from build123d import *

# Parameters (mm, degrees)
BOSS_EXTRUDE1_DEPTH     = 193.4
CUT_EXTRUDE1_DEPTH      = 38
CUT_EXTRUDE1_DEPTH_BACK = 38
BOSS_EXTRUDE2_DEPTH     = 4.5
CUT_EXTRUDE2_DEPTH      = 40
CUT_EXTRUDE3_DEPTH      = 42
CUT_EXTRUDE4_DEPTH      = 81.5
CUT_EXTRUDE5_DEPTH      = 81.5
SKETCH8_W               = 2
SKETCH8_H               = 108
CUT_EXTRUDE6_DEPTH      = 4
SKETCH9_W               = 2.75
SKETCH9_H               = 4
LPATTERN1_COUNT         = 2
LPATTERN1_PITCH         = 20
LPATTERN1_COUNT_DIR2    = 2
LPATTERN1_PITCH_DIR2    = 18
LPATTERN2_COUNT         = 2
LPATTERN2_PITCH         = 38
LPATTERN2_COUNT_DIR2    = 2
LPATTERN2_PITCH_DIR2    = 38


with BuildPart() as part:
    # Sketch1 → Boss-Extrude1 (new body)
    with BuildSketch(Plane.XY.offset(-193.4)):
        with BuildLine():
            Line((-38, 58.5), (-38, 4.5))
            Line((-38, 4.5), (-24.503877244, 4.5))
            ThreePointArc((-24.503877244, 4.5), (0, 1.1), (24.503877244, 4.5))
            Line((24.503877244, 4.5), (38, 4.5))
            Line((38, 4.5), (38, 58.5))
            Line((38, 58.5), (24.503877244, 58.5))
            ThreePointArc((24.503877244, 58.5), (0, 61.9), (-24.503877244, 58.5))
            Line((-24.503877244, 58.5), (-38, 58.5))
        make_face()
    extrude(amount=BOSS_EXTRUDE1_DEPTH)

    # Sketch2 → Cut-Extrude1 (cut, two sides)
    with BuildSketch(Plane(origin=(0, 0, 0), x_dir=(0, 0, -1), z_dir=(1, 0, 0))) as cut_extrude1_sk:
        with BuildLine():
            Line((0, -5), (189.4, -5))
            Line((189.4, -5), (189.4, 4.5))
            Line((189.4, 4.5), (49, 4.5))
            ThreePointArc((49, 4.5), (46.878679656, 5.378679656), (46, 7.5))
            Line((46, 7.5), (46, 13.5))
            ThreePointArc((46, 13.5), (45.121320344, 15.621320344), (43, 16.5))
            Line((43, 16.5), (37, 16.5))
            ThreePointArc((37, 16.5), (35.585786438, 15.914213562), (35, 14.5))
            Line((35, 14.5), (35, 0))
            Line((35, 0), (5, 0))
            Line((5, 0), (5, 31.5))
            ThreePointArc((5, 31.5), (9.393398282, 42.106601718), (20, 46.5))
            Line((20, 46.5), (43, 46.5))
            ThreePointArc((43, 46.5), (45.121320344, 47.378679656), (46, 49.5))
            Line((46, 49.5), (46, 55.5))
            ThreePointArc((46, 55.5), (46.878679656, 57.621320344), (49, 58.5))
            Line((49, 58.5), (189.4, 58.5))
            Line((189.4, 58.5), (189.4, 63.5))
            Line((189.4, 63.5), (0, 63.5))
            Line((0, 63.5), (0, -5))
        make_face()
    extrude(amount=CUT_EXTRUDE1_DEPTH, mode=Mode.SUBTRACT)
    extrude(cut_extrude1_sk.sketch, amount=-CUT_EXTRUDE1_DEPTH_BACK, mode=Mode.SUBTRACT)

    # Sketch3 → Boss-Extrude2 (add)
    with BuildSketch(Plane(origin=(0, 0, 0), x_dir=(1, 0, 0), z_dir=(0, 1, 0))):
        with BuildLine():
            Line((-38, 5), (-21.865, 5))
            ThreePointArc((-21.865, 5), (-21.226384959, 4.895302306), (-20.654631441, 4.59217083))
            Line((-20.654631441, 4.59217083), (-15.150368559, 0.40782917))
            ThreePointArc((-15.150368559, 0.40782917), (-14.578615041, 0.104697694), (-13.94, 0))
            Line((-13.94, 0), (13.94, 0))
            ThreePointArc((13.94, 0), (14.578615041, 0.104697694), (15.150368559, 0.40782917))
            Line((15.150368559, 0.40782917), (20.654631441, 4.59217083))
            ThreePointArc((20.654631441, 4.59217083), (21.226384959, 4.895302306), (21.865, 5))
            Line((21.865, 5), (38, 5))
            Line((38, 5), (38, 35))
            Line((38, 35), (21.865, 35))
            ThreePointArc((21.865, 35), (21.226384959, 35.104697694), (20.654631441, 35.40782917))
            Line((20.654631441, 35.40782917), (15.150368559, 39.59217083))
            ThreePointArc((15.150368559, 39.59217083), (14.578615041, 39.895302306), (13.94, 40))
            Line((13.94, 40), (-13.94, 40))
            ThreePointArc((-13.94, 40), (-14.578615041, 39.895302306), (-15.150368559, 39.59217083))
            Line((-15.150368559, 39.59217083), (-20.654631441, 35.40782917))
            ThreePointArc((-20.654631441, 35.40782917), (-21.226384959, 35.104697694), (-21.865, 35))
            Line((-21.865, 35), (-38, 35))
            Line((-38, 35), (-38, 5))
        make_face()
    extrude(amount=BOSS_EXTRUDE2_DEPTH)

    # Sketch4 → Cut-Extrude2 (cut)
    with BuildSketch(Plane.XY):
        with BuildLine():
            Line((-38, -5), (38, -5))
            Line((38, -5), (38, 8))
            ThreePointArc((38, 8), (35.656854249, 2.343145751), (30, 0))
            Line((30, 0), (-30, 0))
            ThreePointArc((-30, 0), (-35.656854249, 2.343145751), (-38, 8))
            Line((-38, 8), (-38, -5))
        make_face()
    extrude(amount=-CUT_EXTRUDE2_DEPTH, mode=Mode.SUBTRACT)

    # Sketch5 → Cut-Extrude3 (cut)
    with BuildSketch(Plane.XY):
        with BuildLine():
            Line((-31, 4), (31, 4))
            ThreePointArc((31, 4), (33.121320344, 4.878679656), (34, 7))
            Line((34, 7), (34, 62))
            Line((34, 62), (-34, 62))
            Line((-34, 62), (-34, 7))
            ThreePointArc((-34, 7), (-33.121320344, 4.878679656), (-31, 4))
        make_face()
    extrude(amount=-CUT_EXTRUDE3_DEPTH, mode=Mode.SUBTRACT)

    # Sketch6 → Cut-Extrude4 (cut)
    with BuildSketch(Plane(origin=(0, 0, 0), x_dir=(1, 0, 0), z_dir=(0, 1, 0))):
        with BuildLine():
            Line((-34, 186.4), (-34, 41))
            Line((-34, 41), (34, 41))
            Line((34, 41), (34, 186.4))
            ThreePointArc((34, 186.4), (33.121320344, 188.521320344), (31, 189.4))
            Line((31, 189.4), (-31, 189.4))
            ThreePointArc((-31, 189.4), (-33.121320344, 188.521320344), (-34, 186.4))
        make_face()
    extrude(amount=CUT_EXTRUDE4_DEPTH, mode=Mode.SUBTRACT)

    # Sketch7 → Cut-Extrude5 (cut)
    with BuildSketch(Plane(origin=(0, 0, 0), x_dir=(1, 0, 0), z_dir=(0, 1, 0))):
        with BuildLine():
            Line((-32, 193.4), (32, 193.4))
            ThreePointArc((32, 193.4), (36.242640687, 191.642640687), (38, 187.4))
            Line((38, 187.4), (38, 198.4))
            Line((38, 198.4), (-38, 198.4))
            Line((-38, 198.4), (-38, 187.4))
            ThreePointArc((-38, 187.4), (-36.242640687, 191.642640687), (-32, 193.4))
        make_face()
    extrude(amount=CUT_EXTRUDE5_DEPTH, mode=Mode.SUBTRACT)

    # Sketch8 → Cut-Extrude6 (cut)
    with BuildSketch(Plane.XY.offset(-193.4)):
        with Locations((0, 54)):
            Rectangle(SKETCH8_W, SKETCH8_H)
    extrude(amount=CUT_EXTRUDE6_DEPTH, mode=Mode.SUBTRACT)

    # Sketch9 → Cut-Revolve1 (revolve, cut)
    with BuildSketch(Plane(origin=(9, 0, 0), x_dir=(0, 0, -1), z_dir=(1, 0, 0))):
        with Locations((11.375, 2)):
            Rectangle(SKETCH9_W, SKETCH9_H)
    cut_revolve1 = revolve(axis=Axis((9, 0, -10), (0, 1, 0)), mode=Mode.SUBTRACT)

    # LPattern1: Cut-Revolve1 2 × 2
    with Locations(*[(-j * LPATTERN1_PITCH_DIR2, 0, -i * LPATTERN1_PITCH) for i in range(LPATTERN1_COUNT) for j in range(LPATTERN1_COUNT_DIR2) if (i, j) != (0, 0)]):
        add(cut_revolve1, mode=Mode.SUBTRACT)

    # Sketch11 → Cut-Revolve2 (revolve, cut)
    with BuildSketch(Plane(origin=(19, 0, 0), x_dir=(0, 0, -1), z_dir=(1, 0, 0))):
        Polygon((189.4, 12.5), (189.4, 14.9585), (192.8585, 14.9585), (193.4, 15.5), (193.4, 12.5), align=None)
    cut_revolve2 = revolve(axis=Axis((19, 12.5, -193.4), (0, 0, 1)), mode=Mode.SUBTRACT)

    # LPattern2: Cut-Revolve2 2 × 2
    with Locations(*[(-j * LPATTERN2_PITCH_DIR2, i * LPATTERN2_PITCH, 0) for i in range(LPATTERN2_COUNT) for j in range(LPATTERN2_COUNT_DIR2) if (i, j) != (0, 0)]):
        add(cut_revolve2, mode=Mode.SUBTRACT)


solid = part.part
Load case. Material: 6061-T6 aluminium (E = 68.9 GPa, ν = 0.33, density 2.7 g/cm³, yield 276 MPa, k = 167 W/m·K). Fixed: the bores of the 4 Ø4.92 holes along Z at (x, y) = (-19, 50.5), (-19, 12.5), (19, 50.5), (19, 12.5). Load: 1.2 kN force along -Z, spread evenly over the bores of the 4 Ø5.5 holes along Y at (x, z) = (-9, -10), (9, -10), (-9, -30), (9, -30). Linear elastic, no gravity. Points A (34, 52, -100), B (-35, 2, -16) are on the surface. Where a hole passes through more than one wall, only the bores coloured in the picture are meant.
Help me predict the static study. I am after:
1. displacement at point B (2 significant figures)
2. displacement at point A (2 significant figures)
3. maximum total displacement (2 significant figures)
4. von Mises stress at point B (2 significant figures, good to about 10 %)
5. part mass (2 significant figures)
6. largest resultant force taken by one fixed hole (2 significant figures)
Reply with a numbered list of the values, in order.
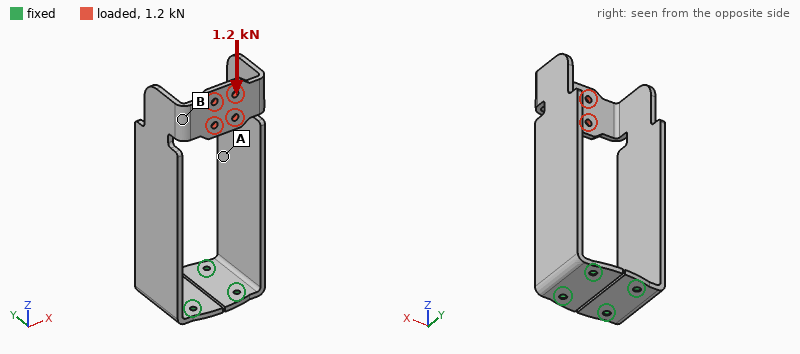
1. 0.51 mm
2. 0.23 mm
3. 0.59 mm
4. 17 MPa
5. 270 g
6. 740 N
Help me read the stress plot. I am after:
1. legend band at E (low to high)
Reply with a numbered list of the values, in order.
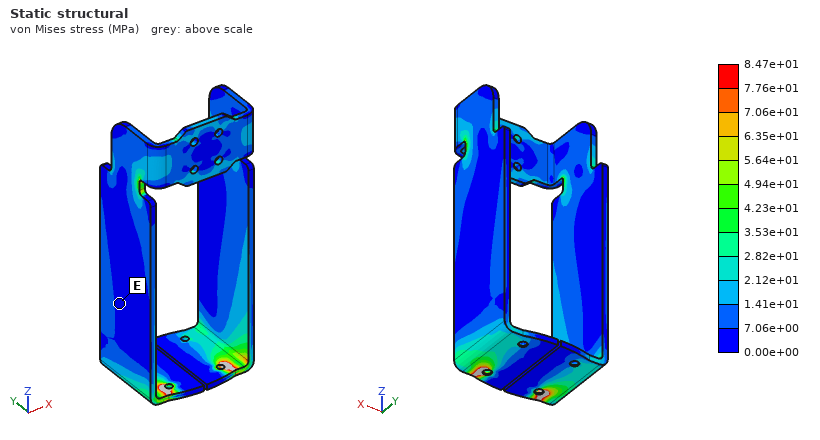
1. 0.00e+00 to 7.06e+00 MPa
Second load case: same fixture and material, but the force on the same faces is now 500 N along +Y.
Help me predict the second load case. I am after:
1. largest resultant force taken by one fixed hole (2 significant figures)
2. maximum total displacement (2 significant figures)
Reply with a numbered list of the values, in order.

1. 1.1 kN
2. 1.5 mm
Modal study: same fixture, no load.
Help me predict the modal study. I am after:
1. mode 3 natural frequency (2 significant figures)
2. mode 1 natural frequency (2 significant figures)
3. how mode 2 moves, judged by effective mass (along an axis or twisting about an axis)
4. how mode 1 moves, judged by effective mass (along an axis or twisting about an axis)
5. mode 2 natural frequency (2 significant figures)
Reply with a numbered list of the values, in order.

1. 460 Hz
2. 110 Hz
3. along Y
4. along X
5. 340 Hz
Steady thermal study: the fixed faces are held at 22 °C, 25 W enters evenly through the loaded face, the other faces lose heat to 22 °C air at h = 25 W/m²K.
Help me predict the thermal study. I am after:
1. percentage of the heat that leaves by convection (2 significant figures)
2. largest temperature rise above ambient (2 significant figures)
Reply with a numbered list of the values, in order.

1. 75 %
2. 51 K
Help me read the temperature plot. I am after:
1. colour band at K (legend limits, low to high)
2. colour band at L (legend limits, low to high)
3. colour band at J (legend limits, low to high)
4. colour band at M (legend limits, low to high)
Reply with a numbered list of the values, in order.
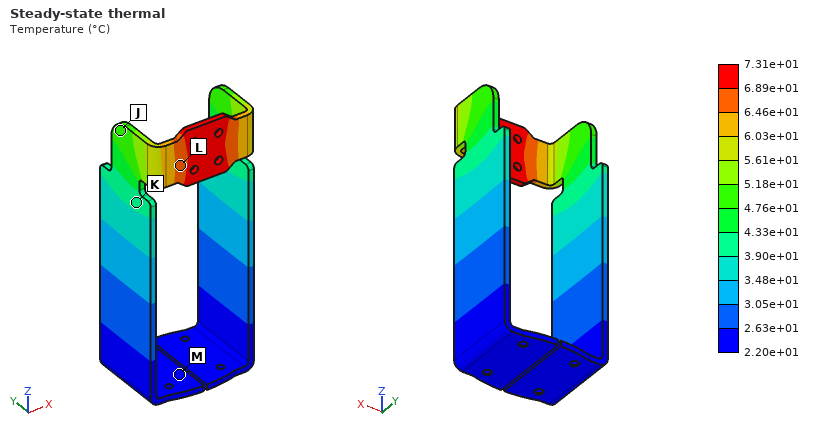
1. 3.90e+01 to 4.33e+01 °C
2. 6.46e+01 to 6.89e+01 °C
3. 4.76e+01 to 5.18e+01 °C
4. 2.20e+01 to 2.63e+01 °C
